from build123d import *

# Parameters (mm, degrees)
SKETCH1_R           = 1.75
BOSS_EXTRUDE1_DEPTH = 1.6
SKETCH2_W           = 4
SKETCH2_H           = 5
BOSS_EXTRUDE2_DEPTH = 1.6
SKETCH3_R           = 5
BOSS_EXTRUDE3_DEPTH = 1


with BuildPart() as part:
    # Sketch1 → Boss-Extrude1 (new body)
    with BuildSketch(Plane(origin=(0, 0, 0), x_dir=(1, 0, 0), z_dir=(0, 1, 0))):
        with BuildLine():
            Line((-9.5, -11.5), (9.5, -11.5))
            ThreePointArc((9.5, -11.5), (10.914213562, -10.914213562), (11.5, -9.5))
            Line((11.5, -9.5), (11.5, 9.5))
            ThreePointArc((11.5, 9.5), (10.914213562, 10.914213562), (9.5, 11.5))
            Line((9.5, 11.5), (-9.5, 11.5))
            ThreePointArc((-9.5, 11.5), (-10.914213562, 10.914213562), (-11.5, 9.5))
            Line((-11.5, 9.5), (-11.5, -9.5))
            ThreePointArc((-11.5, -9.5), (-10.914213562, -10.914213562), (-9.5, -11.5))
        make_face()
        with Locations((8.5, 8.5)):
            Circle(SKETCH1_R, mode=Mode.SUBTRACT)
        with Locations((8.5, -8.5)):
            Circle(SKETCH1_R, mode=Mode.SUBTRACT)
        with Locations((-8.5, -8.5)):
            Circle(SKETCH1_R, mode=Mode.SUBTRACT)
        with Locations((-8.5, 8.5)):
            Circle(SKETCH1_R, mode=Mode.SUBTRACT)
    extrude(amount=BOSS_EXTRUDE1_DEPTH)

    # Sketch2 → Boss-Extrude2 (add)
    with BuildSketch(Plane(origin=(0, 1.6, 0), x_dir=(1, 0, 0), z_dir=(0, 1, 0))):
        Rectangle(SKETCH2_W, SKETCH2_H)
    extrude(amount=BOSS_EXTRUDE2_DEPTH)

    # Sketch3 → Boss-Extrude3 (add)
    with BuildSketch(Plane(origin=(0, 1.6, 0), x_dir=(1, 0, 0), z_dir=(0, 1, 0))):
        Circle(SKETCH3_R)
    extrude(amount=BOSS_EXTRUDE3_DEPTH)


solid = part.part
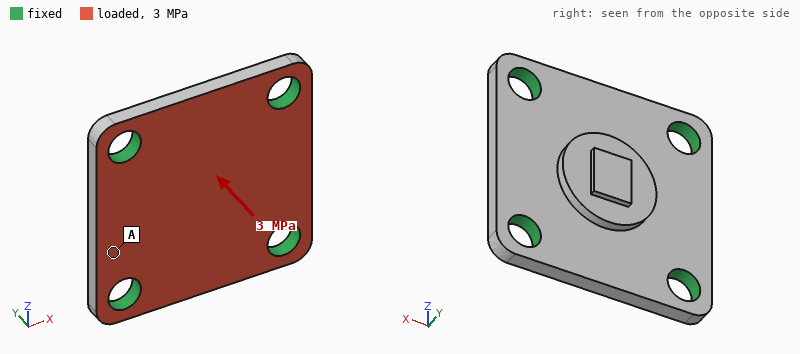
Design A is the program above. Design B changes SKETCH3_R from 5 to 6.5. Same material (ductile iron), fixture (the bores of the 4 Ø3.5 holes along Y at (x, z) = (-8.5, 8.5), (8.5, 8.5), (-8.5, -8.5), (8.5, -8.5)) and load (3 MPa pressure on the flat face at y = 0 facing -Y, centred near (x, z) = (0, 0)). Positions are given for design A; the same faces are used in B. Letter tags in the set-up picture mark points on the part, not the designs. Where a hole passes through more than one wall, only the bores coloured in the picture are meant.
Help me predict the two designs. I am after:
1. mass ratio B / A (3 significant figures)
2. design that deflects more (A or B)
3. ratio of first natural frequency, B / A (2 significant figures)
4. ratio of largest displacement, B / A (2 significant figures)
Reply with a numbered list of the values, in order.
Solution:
1. 1.06
2. A
3. 1.1
4. 0.83
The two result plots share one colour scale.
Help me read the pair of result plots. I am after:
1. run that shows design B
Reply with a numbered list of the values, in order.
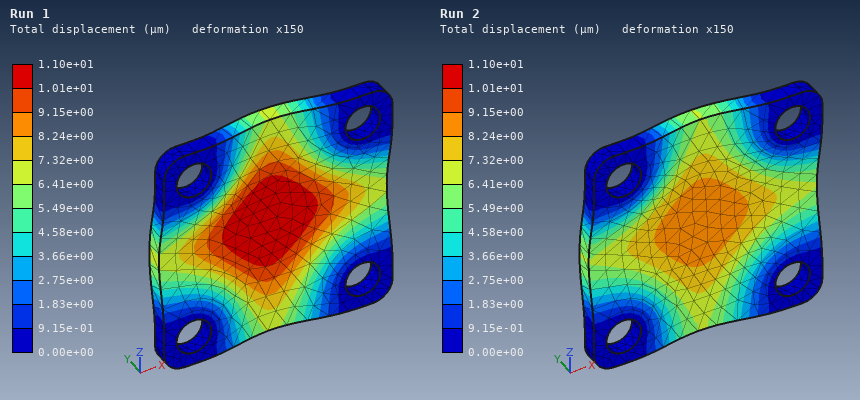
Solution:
1. Run 2
